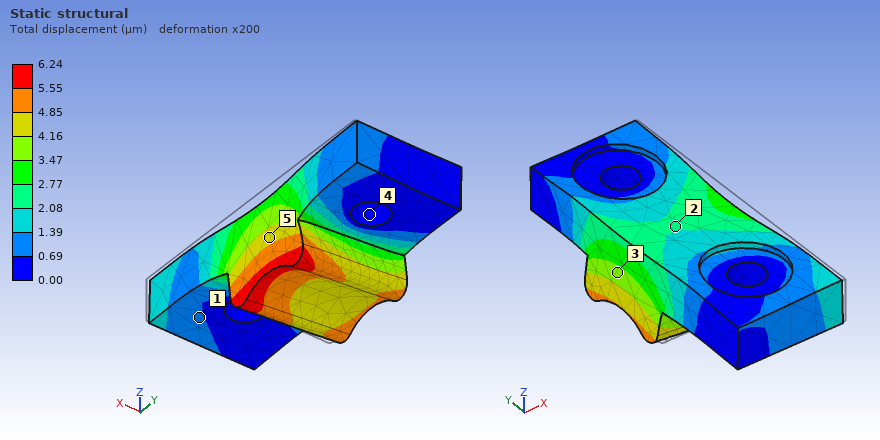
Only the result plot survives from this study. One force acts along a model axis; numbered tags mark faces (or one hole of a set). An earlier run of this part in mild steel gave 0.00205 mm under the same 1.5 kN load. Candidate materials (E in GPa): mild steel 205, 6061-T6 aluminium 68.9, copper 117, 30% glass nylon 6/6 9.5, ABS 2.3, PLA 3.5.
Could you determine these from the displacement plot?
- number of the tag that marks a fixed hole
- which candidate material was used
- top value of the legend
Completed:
4
6061-T6 aluminium
6.24 µm
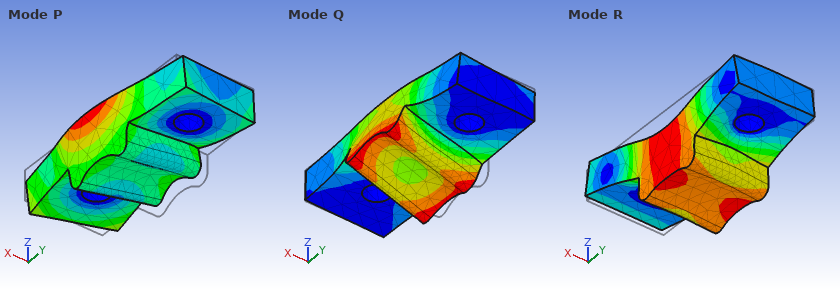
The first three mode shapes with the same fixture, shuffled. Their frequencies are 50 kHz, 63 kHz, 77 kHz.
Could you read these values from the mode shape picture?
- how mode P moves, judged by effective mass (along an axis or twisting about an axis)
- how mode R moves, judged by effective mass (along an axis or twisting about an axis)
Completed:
along X
along Z
